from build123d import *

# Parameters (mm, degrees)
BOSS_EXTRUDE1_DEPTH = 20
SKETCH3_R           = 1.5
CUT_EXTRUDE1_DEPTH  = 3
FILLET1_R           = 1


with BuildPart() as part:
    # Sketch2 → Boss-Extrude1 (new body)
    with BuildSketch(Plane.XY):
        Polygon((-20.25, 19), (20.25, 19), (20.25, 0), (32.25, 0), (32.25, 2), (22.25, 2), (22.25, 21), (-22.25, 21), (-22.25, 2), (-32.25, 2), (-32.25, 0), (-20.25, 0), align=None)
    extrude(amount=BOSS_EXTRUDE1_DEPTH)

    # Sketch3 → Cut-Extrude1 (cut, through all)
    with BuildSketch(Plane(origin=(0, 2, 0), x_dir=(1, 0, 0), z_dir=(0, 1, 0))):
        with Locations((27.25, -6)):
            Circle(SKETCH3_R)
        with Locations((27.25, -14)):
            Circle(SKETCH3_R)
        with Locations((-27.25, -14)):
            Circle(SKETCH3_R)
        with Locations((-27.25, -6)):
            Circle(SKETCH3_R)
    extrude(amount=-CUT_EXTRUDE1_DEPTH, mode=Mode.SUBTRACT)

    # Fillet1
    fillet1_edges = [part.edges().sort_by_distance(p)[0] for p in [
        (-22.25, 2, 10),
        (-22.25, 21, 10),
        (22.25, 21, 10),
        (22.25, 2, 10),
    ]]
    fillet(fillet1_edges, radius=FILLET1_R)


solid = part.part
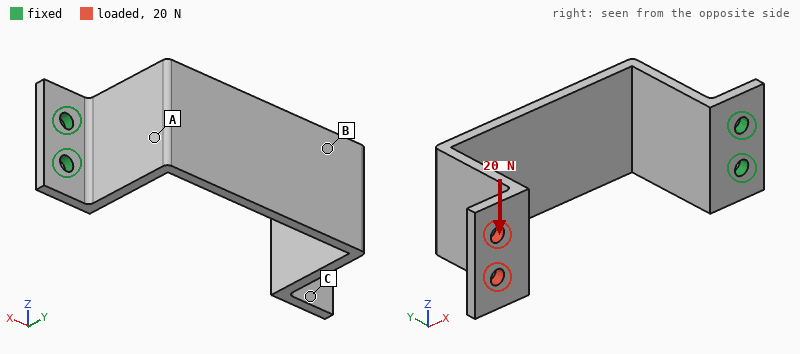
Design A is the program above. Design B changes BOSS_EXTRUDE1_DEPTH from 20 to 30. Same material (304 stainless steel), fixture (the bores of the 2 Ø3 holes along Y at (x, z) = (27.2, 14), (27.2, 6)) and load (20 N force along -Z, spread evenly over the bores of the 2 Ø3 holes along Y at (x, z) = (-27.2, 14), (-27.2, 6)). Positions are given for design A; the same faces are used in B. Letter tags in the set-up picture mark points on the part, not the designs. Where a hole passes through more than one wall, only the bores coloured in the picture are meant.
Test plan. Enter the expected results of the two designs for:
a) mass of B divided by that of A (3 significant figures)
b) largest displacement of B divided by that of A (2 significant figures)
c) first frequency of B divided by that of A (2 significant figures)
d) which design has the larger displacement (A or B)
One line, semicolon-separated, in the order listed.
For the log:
1.51; 0.63; 0.98; A
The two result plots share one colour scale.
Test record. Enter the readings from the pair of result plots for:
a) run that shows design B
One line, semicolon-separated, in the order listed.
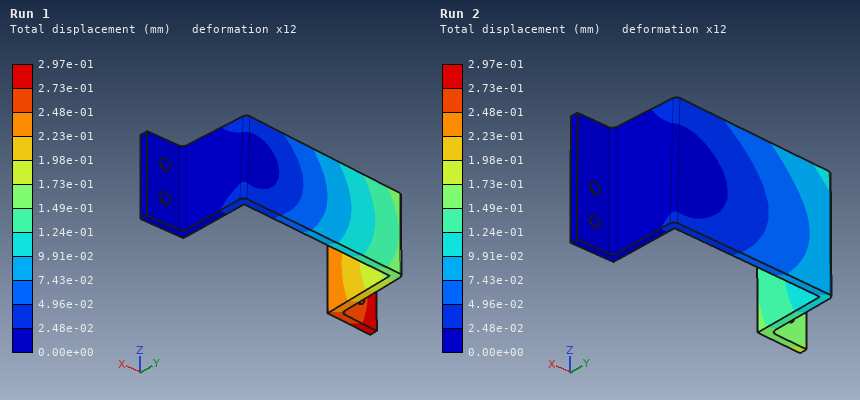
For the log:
Run 2
